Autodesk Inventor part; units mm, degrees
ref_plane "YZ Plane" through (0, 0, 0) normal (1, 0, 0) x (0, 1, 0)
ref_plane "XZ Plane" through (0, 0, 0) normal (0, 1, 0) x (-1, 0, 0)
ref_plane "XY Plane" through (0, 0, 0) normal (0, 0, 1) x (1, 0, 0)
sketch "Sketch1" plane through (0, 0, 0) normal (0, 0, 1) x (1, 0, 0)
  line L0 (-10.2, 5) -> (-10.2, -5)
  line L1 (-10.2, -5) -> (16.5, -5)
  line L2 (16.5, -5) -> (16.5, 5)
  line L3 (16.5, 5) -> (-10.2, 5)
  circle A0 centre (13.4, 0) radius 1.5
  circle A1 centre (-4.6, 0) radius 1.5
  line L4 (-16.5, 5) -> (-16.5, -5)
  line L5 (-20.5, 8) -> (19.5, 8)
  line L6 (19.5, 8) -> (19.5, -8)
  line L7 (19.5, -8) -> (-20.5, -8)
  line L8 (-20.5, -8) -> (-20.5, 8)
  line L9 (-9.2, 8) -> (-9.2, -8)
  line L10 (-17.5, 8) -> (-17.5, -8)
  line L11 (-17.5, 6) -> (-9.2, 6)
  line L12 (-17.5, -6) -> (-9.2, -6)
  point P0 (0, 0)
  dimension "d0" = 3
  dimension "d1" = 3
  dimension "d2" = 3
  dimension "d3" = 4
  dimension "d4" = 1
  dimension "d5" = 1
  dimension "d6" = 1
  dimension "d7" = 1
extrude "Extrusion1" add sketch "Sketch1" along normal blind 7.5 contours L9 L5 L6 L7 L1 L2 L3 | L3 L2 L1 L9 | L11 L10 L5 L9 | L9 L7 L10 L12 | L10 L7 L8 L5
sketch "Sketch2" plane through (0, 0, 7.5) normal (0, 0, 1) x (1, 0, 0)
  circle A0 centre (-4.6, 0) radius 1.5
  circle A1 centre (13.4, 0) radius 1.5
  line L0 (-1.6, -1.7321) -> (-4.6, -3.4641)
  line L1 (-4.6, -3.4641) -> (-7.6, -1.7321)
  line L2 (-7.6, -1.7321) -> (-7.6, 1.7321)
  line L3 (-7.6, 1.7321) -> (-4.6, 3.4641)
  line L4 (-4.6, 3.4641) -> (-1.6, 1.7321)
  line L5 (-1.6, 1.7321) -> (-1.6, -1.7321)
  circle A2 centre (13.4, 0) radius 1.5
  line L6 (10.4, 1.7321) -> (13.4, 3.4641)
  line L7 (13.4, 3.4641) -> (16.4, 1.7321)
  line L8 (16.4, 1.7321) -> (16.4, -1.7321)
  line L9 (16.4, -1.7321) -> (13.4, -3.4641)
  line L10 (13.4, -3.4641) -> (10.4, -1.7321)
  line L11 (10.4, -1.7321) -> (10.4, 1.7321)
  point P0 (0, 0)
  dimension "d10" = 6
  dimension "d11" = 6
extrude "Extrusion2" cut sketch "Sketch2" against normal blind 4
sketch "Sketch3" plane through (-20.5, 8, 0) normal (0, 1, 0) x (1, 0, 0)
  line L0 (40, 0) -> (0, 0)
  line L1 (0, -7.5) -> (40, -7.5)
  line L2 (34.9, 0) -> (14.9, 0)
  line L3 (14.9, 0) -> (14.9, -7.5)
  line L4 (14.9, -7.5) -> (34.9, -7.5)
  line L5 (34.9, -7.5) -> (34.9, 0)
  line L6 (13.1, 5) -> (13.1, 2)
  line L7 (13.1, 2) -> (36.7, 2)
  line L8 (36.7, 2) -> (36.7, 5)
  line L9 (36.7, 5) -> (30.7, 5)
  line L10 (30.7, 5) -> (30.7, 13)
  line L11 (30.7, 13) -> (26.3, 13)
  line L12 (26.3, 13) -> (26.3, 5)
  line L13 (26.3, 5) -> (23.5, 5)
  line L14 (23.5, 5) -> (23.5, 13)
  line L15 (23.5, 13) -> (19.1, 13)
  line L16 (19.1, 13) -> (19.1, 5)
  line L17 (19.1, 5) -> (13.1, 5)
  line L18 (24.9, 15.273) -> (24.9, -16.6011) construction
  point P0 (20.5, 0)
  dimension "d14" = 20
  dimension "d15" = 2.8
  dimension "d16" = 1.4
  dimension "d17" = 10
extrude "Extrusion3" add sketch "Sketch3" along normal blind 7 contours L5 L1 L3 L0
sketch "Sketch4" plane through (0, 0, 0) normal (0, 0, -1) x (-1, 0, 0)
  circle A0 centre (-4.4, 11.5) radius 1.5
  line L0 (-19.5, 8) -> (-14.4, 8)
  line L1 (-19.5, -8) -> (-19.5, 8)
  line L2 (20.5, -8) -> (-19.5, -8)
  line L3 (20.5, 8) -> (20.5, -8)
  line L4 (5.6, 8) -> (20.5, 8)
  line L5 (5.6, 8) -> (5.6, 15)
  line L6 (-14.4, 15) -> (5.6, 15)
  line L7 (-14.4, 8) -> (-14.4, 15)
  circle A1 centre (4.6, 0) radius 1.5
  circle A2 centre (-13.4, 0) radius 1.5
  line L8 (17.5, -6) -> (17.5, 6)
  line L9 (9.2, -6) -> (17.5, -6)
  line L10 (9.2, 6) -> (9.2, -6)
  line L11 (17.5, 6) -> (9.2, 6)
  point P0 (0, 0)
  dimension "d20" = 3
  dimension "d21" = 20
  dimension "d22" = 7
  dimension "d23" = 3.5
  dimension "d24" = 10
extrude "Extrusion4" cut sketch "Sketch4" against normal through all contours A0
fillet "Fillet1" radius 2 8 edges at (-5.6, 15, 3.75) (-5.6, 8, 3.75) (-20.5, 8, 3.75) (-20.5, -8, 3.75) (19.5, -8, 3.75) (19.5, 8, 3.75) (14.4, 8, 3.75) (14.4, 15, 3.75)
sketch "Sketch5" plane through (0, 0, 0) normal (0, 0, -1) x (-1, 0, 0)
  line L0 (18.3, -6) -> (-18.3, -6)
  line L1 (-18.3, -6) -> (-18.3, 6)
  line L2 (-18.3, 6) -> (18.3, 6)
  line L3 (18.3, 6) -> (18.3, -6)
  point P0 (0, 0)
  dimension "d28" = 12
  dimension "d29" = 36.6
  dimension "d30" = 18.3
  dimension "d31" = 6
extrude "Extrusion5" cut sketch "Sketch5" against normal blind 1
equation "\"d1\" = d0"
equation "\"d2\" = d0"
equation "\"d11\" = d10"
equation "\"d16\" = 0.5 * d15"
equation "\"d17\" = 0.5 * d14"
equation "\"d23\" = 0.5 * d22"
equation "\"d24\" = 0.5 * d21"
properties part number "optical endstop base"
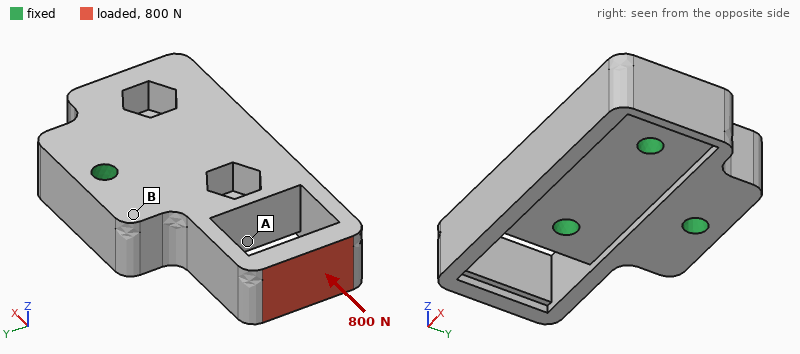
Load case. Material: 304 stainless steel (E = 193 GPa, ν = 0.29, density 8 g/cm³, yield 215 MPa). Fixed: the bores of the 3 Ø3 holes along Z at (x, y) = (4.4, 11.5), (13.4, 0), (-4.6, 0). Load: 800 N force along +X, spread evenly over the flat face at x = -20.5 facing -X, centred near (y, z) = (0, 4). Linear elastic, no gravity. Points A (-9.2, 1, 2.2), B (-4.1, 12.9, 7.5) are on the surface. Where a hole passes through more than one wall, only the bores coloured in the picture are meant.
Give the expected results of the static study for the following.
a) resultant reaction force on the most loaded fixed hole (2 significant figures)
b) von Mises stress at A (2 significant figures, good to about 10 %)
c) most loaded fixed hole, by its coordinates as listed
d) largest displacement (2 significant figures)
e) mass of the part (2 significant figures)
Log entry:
360 N
19 MPa
(-4.6, 0)
10 µm
35 g
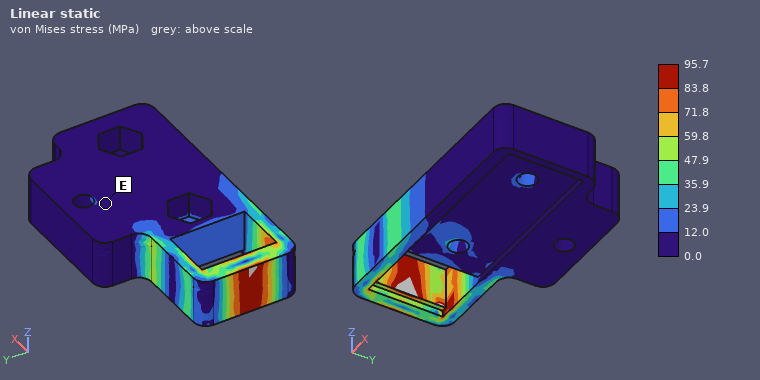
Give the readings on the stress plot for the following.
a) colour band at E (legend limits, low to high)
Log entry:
0.0 to 12.0 MPa
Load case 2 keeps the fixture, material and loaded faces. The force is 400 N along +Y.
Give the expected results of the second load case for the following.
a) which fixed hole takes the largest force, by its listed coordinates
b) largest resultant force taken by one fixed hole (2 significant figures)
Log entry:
(-4.6, 0)
520 N
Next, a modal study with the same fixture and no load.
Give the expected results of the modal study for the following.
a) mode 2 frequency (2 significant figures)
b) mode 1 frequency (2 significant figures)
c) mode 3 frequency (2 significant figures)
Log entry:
12 kHz
11 kHz
18 kHz
